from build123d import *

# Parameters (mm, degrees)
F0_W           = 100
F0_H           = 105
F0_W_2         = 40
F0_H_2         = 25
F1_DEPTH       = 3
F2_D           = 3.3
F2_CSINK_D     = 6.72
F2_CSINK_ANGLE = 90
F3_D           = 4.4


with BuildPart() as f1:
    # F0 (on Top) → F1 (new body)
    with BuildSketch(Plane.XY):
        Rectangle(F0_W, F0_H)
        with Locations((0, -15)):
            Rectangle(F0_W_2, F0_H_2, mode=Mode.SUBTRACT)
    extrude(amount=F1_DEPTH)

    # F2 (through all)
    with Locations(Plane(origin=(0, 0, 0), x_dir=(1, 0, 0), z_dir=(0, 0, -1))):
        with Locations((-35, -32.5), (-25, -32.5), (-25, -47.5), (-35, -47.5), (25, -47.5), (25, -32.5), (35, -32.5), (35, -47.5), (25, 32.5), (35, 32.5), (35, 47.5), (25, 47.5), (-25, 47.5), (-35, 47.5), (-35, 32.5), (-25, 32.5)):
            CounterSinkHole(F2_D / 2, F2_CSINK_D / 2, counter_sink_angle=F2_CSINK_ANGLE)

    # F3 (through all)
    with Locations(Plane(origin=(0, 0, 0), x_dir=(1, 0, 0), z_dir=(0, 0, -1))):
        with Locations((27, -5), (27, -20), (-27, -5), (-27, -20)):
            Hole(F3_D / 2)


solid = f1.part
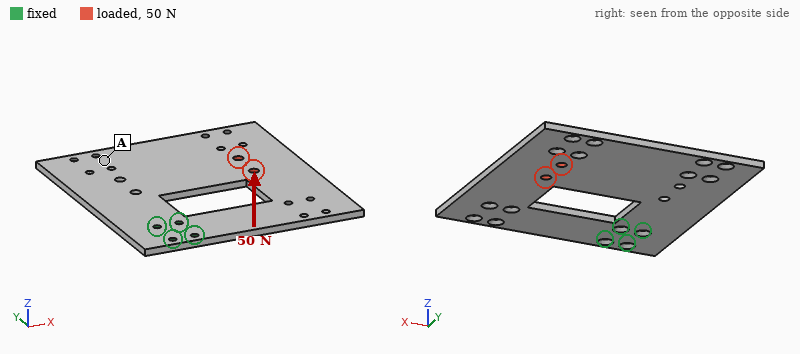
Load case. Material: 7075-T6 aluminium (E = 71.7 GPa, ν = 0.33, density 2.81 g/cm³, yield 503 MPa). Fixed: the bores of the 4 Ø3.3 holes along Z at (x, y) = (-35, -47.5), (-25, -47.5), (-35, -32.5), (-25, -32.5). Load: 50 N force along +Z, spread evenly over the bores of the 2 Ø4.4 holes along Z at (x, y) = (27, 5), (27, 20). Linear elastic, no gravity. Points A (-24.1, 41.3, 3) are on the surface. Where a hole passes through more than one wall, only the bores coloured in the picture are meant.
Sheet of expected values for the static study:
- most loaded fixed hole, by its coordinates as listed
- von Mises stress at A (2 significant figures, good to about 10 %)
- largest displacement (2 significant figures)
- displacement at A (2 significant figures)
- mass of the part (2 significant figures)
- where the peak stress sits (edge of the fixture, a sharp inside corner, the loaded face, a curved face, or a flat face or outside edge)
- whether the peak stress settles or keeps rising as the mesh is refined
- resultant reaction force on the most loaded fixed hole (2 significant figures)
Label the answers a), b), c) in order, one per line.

a) (-25, -32.5)
b) 8.6 MPa
c) 1.6 mm
d) 0.58 mm
e) 78 g
f) edge of the fixture
g) keeps rising
h) 290 N
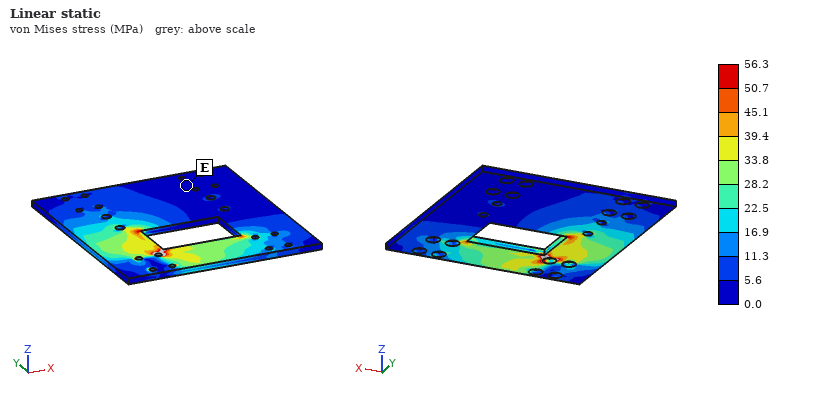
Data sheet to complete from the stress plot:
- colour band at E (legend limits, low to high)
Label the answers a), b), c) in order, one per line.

a) 0.0 to 5.6 MPa
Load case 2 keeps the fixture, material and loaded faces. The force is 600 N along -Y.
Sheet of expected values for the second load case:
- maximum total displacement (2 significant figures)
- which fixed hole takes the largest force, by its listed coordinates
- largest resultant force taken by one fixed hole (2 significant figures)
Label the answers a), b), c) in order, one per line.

a) 0.13 mm
b) (-25, -32.5)
c) 1.3 kN
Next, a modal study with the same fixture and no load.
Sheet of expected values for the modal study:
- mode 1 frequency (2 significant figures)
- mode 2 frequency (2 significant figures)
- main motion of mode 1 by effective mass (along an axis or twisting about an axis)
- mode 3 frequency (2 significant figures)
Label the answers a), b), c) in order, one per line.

a) 180 Hz
b) 350 Hz
c) along Z
d) 760 Hz
